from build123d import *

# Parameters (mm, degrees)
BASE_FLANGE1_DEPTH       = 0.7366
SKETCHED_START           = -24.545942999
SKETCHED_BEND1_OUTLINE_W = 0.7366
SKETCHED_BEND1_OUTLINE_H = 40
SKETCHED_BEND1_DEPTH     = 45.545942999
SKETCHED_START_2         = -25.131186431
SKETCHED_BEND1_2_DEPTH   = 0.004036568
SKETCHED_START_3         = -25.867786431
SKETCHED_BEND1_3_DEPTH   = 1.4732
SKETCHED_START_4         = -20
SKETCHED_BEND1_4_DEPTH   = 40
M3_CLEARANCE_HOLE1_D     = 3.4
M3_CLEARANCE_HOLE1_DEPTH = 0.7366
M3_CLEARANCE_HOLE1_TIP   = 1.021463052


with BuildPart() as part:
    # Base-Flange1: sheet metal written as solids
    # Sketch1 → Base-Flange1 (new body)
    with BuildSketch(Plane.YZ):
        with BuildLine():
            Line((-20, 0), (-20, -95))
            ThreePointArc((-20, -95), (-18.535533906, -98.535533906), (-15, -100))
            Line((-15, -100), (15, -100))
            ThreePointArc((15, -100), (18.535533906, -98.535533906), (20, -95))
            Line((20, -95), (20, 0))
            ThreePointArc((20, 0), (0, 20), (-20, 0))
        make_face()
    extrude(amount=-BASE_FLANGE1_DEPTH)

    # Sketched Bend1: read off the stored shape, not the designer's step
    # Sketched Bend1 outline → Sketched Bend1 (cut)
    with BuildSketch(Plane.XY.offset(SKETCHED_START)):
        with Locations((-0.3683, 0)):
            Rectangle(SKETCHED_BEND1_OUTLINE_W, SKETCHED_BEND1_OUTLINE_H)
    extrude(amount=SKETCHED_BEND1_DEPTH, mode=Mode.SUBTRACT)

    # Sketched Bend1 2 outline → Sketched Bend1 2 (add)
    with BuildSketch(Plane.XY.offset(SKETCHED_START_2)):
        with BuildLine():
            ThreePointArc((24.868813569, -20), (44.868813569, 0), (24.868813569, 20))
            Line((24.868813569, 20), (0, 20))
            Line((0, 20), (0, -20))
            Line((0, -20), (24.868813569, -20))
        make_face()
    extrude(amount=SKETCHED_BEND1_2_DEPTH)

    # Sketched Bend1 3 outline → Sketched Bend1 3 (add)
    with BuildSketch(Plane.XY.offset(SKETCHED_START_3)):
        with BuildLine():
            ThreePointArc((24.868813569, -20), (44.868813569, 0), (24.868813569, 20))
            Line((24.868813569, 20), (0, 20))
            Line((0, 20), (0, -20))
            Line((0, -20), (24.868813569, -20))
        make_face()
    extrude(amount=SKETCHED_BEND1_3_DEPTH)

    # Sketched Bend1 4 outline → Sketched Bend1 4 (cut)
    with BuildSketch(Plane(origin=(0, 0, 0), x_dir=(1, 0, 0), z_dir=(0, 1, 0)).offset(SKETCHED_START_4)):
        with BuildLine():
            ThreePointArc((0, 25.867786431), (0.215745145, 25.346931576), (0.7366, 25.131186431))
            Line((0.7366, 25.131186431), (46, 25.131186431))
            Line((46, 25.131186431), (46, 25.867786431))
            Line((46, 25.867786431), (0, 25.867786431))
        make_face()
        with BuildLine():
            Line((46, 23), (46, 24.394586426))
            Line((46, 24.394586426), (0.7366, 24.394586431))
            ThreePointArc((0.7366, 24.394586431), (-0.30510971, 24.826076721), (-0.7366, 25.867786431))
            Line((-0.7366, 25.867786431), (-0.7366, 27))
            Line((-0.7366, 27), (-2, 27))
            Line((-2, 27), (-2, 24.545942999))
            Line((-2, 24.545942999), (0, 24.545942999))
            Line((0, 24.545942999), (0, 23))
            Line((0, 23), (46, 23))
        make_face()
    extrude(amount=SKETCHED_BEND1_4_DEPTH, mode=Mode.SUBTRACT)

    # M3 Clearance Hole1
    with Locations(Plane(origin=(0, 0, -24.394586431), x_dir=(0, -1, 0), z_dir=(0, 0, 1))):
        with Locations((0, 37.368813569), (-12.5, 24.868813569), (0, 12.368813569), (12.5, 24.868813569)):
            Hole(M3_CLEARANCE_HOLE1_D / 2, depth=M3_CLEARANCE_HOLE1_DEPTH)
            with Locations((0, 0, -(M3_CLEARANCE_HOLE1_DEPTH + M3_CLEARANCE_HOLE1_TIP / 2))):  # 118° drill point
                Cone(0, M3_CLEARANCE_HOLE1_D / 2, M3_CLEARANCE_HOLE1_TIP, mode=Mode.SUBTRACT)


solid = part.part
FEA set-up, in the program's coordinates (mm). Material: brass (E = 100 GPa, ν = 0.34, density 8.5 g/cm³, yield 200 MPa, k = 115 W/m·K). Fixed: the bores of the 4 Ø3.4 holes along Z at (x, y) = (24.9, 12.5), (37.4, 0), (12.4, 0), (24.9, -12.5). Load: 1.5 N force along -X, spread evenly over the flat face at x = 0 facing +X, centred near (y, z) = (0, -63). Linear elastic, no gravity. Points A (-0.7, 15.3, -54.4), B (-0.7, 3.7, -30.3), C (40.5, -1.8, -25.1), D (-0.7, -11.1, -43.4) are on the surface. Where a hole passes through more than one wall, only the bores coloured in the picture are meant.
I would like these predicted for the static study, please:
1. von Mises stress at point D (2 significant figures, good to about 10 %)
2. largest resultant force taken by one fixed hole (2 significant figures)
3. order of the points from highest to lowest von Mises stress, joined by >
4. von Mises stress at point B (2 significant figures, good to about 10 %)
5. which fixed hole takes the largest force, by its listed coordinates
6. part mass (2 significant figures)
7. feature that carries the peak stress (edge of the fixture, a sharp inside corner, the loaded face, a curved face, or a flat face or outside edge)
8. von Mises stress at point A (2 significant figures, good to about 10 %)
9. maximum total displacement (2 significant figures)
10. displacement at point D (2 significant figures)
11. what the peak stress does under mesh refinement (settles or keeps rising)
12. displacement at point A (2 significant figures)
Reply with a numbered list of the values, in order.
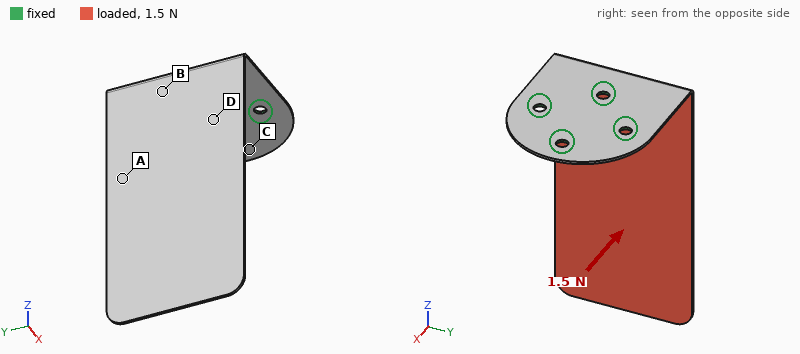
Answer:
1. 8.3 MPa
2. 2.5 N
3. B > D > A > C
4. 12 MPa
5. (12.4, 0)
6. 29 g
7. edge of the fixture
8. 5.8 MPa
9. 0.96 mm
10. 0.16 mm
11. keeps rising
12. 0.29 mm
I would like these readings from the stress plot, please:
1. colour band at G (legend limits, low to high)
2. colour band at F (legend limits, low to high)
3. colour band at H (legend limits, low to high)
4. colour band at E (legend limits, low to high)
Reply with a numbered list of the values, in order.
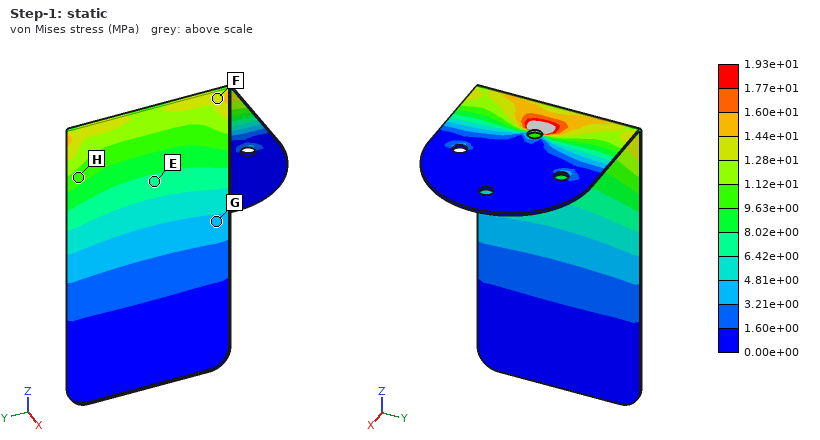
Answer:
1. 3.21e+00 to 4.81e+00 MPa
2. 1.28e+01 to 1.44e+01 MPa
3. 9.63e+00 to 1.12e+01 MPa
4. 6.42e+00 to 8.02e+00 MPa
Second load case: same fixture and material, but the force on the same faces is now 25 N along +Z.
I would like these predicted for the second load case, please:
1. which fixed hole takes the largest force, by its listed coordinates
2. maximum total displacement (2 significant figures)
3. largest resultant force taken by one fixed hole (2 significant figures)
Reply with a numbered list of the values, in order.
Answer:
1. (12.4, 0)
2. 1.1 mm
3. 32 N
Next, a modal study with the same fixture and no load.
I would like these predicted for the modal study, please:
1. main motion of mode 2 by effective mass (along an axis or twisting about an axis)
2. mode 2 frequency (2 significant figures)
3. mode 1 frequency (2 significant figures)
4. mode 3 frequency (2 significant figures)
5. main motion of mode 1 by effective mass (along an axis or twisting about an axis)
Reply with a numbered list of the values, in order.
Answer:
1. along Y
2. 120 Hz
3. 58 Hz
4. 290 Hz
5. along X
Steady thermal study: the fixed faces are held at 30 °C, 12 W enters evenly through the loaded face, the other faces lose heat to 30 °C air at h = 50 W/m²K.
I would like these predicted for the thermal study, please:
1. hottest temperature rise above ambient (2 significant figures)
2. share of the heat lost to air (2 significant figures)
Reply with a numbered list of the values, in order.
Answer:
1. 60 K
2. 70 %
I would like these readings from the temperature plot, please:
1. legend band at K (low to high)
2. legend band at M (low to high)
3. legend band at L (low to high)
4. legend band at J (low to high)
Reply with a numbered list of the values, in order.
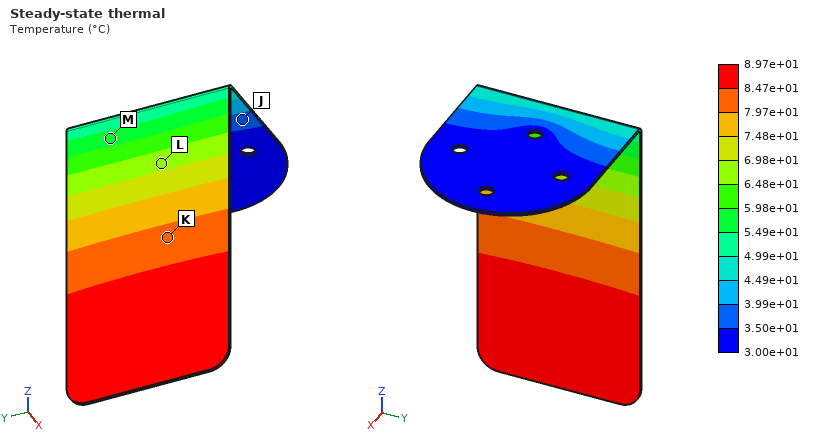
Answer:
1. 7.97e+01 to 8.47e+01 °C
2. 5.49e+01 to 5.98e+01 °C
3. 6.48e+01 to 6.98e+01 °C
4. 3.50e+01 to 3.99e+01 °C
